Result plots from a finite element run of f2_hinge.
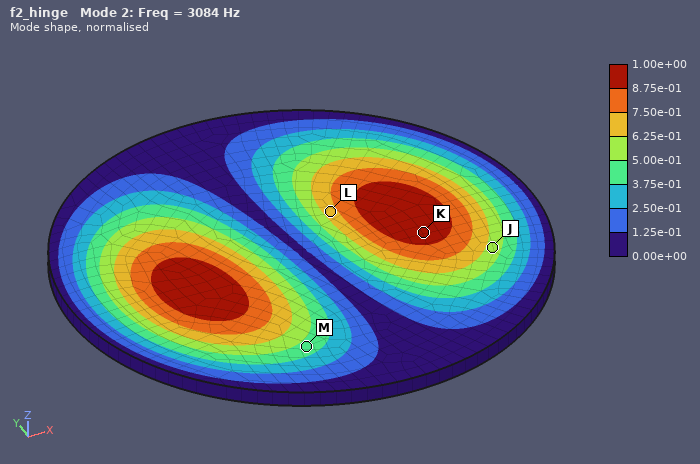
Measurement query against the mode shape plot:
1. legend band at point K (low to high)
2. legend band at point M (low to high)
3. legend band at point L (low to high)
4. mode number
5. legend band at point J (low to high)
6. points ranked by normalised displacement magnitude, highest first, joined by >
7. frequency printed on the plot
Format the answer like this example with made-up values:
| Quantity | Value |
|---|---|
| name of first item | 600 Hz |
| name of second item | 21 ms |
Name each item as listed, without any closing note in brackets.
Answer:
| Quantity | Value |
|---|---|
| legend band at point K | 8.75e-01 to 1.00e+00 |
| legend band at point M | 3.75e-01 to 5.00e-01 |
| legend band at point L | 6.25e-01 to 7.50e-01 |
| mode number | 2 |
| legend band at point J | 5.00e-01 to 6.25e-01 |
| points ranked by normalised displacement magnitude, highest first, joined by > | K > L > J > M |
| frequency printed on the plot | 3084 Hz |
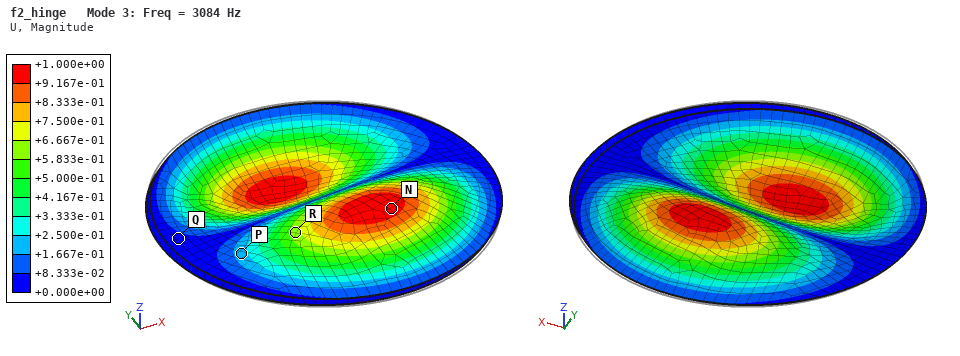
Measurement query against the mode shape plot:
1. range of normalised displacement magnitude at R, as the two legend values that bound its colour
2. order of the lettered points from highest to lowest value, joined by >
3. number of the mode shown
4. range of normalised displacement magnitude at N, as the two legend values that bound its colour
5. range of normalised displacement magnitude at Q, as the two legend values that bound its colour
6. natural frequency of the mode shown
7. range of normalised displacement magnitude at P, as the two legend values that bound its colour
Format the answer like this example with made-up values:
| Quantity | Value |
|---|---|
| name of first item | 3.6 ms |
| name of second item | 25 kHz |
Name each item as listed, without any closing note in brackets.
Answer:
| Quantity | Value |
|---|---|
| range of normalised displacement magnitude at R, as the two legend values that bound its colour | +5.833e-01 to +6.667e-01 |
| order of the lettered points from highest to lowest value, joined by > | N > R > P > Q |
| number of the mode shown | 3 |
| range of normalised displacement magnitude at N, as the two legend values that bound its colour | +9.167e-01 to +1.000e+00 |
| range of normalised displacement magnitude at Q, as the two legend values that bound its colour | +0.000e+00 to +8.333e-02 |
| natural frequency of the mode shown | 3084 Hz |
| range of normalised displacement magnitude at P, as the two legend values that bound its colour | +1.667e-01 to +2.500e-01 |
